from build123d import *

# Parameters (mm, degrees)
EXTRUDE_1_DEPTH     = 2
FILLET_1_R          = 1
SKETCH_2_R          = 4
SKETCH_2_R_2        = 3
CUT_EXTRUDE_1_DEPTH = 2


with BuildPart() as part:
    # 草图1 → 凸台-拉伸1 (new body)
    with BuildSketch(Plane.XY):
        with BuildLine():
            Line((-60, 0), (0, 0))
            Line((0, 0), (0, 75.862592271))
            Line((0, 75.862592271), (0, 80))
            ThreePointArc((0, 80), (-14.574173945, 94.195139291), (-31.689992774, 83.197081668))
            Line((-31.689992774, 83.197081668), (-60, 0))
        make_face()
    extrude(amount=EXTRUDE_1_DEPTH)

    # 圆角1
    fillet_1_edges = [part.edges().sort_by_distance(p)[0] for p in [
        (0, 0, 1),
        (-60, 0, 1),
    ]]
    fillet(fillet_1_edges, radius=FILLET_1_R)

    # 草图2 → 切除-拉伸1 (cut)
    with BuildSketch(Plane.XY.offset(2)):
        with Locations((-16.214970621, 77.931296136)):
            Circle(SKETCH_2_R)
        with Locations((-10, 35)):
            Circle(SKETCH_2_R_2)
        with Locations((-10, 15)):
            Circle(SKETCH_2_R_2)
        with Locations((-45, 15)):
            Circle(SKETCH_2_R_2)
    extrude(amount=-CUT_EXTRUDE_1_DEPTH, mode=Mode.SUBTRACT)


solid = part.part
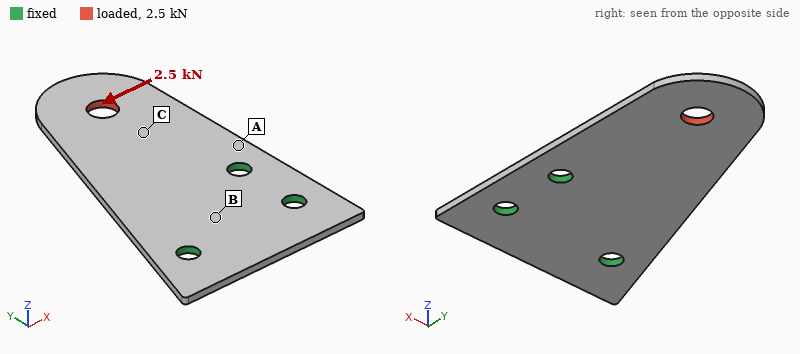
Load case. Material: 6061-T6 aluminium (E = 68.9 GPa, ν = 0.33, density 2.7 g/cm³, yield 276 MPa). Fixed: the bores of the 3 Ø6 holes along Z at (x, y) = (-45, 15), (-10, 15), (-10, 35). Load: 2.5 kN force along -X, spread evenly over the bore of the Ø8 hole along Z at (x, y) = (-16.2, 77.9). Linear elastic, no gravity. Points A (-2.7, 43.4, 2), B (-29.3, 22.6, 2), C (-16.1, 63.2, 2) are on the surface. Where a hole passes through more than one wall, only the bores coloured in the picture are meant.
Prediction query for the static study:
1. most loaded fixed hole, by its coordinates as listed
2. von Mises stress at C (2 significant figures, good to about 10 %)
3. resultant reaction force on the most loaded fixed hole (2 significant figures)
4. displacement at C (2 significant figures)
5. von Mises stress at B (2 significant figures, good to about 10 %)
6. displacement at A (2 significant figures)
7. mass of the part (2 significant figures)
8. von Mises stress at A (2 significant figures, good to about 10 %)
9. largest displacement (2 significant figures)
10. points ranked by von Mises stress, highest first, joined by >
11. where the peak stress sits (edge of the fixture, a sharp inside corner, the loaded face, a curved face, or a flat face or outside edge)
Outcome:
(-10, 35)
76 MPa
3.6 kN
0.094 mm
22 MPa
0.036 mm
21 g
110 MPa
0.23 mm
A > C > B
edge of the fixture
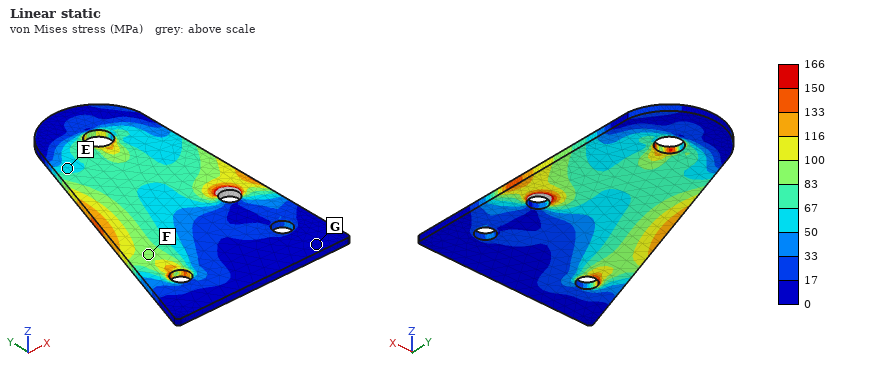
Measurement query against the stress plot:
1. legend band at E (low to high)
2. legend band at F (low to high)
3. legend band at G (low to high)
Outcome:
50 to 67 MPa
83 to 100 MPa
0 to 17 MPa
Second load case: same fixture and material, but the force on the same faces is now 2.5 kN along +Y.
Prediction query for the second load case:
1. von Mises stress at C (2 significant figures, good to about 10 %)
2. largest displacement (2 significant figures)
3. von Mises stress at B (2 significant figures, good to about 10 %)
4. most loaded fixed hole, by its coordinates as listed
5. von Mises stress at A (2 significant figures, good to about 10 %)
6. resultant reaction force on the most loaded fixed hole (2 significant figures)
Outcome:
45 MPa
35 µm
7.5 MPa
(-10, 35)
40 MPa
1.6 kN
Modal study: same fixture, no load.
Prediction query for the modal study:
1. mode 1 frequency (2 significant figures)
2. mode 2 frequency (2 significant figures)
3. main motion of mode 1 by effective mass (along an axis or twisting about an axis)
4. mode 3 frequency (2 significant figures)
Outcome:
580 Hz
1700 Hz
along Z
3000 Hz
